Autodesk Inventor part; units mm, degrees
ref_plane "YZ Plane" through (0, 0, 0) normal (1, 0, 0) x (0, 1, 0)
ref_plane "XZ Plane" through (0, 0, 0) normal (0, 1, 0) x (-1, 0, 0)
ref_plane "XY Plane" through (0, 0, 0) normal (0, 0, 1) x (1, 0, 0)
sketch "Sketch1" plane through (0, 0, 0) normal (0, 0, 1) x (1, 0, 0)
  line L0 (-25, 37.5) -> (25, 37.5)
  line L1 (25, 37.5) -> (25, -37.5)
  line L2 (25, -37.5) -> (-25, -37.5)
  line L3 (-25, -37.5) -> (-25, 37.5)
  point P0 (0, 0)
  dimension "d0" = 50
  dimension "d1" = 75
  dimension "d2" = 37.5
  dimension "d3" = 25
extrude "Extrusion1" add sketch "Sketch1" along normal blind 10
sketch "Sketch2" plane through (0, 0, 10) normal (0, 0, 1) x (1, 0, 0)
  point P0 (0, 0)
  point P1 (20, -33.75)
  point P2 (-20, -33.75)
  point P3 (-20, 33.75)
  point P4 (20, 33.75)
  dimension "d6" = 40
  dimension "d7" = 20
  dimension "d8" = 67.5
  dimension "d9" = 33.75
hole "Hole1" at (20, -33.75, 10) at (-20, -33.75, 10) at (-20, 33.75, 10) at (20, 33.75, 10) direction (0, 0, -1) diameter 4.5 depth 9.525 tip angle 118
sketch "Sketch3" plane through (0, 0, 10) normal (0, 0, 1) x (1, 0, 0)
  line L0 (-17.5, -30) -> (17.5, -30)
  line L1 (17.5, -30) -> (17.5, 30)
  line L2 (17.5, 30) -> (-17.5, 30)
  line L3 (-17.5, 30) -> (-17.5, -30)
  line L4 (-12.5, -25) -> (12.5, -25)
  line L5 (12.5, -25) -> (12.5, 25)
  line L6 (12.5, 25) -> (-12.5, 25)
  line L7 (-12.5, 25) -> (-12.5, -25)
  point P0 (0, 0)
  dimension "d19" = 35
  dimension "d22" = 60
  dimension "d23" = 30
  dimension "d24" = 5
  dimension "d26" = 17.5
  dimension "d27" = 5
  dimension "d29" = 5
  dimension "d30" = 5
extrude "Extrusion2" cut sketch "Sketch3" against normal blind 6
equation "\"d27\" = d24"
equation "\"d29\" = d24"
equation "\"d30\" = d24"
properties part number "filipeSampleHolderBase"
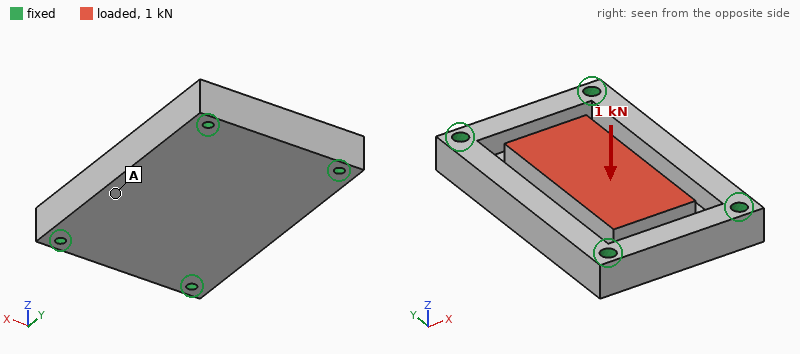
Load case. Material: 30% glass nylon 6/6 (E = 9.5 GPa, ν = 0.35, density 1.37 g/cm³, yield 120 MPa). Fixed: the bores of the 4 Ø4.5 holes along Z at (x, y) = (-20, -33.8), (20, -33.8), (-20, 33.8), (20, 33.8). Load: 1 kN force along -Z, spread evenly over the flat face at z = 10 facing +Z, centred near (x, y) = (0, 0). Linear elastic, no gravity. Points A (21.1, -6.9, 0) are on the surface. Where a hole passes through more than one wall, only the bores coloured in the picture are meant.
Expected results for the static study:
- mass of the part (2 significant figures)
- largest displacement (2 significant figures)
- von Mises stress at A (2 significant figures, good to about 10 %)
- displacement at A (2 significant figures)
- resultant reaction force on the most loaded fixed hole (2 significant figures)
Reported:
44 g
71 µm
5.2 MPa
44 µm
250 N
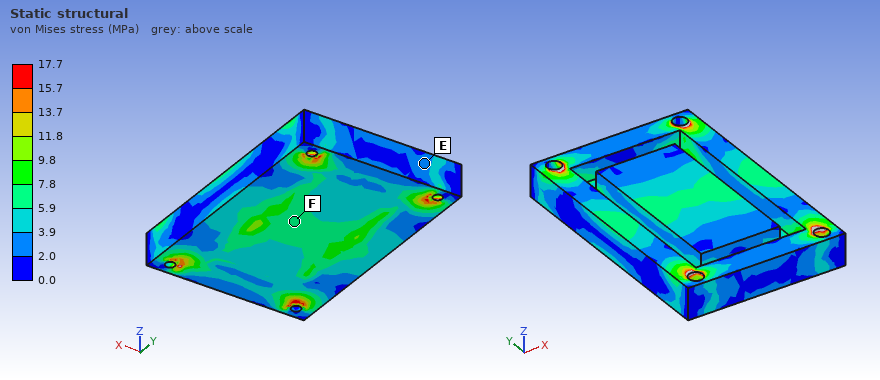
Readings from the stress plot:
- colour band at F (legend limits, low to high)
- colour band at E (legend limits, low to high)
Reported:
5.9 to 7.8 MPa
2.0 to 3.9 MPa
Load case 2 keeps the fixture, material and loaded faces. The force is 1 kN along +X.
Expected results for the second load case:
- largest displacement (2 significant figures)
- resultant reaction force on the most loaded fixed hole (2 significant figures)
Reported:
36 µm
300 N
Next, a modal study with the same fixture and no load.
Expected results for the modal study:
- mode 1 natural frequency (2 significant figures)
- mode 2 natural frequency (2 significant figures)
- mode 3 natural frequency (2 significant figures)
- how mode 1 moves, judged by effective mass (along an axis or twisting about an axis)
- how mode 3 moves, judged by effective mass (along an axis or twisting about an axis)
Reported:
4100 Hz
5800 Hz
8200 Hz
along Z
along X
